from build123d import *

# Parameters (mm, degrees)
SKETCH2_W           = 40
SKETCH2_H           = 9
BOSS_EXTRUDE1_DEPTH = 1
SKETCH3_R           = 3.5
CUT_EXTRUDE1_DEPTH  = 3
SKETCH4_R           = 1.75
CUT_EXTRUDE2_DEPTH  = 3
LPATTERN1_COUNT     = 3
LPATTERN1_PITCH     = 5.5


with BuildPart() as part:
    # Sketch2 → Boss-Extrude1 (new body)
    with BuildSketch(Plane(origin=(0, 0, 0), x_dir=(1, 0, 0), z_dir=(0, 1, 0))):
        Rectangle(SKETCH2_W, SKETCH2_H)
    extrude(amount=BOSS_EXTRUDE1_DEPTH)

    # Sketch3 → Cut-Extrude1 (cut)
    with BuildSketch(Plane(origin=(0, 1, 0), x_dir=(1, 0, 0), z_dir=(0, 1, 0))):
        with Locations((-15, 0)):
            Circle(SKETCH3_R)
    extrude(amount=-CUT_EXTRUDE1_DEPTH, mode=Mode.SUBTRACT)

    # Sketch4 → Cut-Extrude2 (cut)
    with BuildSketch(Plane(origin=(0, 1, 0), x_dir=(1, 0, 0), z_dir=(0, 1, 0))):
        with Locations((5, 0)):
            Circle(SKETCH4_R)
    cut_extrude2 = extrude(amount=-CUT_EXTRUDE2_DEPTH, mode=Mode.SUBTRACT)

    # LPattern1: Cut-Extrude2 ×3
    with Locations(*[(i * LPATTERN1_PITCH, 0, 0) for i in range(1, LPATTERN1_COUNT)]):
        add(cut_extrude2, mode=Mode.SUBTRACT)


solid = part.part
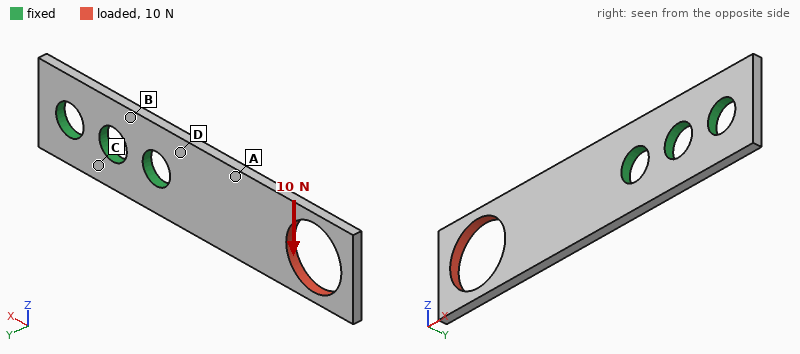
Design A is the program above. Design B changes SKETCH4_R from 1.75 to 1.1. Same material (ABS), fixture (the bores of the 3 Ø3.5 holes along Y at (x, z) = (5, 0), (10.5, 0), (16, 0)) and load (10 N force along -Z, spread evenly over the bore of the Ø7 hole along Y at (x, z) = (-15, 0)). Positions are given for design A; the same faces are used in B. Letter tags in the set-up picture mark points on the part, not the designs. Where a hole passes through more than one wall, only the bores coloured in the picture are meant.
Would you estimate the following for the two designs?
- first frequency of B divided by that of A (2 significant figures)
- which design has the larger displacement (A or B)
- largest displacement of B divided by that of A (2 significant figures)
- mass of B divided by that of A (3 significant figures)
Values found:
0.93
B
1.1
1.06
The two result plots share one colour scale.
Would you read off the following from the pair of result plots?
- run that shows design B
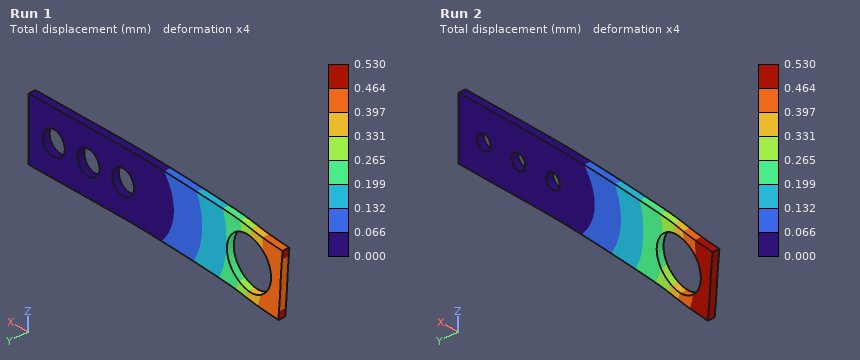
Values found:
Run 2
